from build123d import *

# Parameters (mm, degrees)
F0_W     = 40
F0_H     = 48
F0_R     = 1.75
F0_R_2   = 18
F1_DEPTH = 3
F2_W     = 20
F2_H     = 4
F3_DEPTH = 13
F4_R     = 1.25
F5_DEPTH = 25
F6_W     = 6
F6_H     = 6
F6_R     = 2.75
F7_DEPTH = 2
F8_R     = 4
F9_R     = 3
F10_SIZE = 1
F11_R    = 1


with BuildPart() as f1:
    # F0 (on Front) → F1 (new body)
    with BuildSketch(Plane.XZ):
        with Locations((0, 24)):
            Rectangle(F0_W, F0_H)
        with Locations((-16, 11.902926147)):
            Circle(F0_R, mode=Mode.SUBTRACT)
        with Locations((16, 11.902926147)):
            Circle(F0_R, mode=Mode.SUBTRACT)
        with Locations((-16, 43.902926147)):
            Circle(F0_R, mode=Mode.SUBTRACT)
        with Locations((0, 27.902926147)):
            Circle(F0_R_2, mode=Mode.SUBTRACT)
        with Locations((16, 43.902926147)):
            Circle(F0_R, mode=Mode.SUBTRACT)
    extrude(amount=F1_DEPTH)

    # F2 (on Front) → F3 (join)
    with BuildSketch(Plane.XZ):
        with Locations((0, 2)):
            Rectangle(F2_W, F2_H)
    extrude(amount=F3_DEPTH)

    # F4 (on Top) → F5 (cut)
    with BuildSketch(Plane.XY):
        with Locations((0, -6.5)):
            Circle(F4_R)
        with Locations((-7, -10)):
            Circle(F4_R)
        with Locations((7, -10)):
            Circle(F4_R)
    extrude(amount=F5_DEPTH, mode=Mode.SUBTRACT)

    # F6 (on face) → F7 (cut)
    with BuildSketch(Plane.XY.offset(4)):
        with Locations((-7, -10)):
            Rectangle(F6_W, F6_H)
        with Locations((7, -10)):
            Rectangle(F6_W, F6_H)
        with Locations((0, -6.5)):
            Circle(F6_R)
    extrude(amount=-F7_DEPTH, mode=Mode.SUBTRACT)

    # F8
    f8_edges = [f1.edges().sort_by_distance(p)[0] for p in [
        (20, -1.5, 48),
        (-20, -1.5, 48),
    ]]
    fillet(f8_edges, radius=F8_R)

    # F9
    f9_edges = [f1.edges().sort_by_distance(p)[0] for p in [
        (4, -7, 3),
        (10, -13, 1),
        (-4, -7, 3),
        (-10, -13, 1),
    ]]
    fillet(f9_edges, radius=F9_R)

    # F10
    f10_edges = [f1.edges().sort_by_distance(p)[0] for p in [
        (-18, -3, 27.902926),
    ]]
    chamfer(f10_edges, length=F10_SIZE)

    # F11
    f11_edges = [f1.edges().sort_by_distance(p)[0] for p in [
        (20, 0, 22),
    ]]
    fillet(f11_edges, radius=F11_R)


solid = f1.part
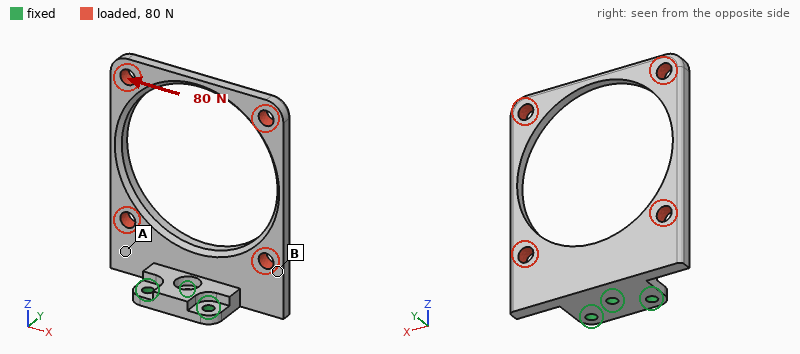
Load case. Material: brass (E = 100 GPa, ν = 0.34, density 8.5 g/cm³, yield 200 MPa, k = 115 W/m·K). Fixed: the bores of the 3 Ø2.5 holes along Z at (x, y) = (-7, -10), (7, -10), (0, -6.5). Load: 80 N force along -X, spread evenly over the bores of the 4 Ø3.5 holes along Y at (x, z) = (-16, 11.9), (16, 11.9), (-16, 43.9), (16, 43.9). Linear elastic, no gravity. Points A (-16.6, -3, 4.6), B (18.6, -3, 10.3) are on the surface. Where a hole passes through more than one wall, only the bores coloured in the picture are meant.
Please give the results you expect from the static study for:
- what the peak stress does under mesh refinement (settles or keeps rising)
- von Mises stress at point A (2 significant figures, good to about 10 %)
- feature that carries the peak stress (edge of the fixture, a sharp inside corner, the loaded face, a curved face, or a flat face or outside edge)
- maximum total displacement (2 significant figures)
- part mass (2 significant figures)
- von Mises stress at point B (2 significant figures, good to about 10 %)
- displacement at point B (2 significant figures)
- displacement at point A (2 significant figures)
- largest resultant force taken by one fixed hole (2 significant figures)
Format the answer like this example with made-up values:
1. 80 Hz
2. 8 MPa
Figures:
1. keeps rising
2. 4.6 MPa
3. edge of the fixture
4. 92 µm
5. 26 g
6. 8.5 MPa
7. 21 µm
8. 15 µm
9. 140 N
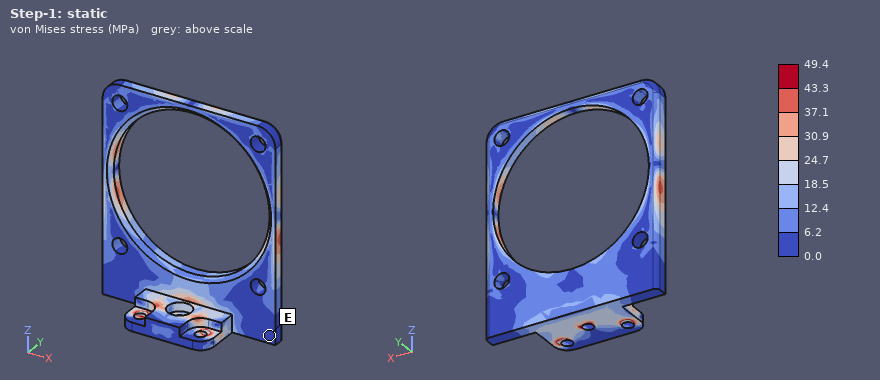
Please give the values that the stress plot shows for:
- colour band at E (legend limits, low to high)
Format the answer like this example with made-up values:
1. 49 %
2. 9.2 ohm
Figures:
1. 0.0 to 6.2 MPa
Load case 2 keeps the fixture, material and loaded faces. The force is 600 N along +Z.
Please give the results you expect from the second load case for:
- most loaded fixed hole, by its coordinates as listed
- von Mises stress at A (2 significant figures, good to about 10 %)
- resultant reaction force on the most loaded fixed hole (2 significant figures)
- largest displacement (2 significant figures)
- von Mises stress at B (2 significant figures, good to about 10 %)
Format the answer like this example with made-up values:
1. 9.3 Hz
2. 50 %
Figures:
1. (0, -6.5)
2. 17 MPa
3. 690 N
4. 0.14 mm
5. 25 MPa
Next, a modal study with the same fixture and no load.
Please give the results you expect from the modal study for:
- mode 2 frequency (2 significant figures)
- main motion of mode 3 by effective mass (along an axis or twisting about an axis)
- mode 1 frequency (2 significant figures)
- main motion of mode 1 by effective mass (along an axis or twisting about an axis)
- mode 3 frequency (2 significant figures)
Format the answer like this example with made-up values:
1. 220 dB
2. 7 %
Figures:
1. 1200 Hz
2. along X
3. 560 Hz
4. along Y
5. 1500 Hz
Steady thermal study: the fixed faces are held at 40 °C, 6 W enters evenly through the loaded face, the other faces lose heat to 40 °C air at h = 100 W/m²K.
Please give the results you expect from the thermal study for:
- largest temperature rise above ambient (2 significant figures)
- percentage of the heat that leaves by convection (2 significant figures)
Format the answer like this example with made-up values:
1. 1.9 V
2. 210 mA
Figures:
1. 25 K
2. 50 %
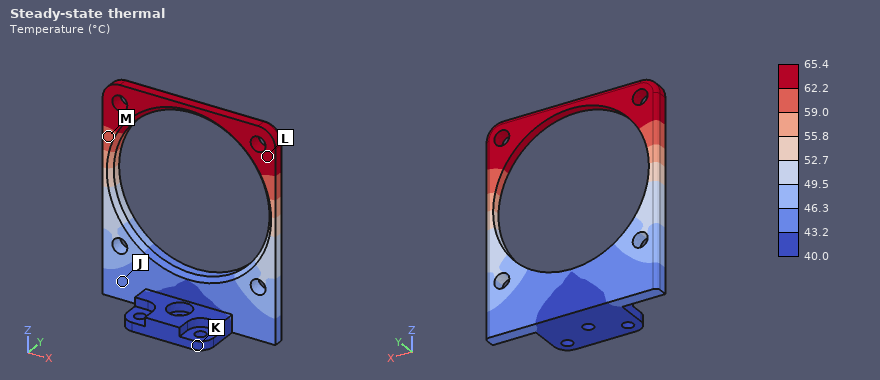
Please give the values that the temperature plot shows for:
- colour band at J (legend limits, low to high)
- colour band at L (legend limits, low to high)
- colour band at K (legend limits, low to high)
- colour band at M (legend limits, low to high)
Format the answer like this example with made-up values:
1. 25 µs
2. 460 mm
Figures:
1. 43.2 to 46.3 °C
2. 62.2 to 65.4 °C
3. 40.0 to 43.2 °C
4. 59.0 to 62.2 °C
